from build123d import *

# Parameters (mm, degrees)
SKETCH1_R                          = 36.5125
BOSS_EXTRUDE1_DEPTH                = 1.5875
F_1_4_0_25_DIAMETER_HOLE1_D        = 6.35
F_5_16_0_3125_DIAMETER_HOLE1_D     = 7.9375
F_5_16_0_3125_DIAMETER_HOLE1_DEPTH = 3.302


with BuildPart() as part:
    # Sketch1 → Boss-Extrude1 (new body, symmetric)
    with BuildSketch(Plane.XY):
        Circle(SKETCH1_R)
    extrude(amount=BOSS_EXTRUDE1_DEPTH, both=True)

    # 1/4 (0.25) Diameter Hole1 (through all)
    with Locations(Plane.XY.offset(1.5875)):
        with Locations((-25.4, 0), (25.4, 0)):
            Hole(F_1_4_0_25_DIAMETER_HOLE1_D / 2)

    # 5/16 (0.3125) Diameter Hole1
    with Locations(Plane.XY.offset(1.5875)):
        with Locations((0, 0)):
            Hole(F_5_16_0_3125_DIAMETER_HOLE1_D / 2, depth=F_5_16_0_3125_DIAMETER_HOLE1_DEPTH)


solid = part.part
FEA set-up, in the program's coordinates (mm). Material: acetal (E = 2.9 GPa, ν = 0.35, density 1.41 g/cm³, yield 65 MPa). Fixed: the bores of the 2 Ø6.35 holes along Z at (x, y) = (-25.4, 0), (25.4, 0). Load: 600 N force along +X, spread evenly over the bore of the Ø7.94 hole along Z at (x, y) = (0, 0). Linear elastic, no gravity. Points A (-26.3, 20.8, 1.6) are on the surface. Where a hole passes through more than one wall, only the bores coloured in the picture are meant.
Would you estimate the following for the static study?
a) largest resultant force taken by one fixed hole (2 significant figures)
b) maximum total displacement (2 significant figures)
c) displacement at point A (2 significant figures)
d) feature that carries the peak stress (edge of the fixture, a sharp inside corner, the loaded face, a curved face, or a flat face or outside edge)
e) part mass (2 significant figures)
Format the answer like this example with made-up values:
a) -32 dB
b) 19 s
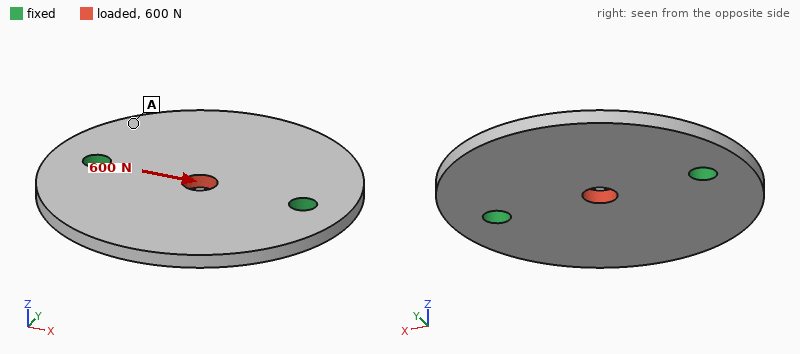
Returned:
a) 300 N
b) 45 µm
c) 19 µm
d) the loaded face
e) 18 g
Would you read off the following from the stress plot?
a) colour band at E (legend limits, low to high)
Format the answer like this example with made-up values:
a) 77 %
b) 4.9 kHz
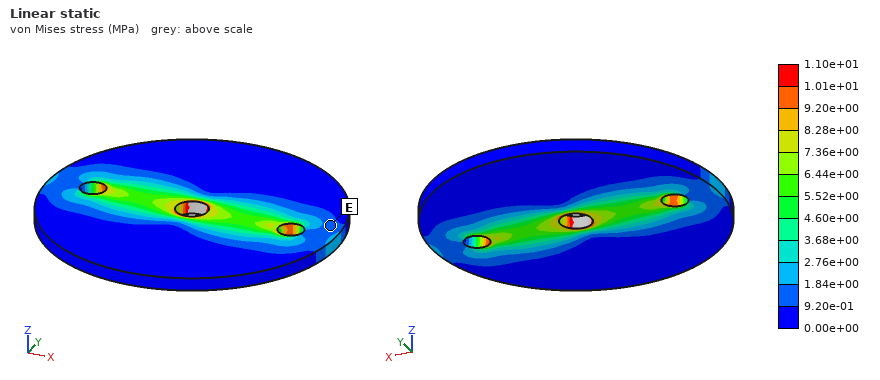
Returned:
a) 9.20e-01 to 1.84e+00 MPa
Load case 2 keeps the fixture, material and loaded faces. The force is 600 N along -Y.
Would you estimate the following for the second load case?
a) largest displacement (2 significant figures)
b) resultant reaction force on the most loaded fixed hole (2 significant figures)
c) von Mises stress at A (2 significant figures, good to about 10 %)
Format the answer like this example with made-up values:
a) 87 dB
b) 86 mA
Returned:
a) 63 µm
b) 300 N
c) 1.5 MPa
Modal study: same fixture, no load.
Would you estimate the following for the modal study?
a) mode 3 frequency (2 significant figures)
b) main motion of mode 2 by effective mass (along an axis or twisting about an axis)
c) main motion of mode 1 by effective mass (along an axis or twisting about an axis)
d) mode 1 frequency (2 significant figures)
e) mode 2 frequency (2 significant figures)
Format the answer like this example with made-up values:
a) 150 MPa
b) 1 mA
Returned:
a) 1500 Hz
b) along Z
c) twisting about X
d) 600 Hz
e) 720 Hz
